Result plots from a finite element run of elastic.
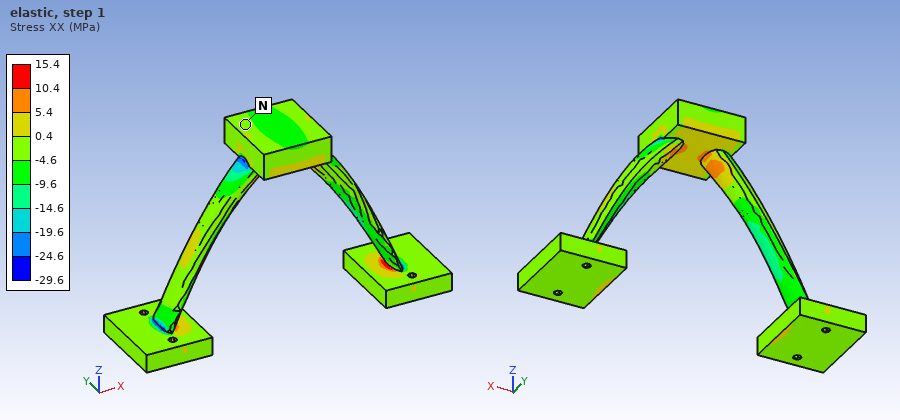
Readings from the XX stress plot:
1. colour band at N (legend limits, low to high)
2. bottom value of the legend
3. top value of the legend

-4.6 to 0.4 MPa
-29.6 MPa
15.4 MPa
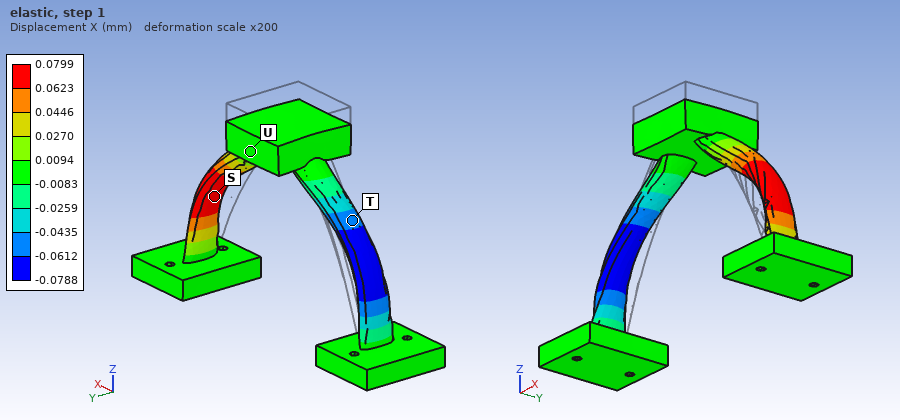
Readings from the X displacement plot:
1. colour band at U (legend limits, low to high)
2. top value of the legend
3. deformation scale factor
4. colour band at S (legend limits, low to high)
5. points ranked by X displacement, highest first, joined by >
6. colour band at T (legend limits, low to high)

-0.0083 to 0.0094 mm
0.0799 mm
200
0.0623 to 0.0799 mm
S > U > T
-0.0612 to -0.0435 mm
